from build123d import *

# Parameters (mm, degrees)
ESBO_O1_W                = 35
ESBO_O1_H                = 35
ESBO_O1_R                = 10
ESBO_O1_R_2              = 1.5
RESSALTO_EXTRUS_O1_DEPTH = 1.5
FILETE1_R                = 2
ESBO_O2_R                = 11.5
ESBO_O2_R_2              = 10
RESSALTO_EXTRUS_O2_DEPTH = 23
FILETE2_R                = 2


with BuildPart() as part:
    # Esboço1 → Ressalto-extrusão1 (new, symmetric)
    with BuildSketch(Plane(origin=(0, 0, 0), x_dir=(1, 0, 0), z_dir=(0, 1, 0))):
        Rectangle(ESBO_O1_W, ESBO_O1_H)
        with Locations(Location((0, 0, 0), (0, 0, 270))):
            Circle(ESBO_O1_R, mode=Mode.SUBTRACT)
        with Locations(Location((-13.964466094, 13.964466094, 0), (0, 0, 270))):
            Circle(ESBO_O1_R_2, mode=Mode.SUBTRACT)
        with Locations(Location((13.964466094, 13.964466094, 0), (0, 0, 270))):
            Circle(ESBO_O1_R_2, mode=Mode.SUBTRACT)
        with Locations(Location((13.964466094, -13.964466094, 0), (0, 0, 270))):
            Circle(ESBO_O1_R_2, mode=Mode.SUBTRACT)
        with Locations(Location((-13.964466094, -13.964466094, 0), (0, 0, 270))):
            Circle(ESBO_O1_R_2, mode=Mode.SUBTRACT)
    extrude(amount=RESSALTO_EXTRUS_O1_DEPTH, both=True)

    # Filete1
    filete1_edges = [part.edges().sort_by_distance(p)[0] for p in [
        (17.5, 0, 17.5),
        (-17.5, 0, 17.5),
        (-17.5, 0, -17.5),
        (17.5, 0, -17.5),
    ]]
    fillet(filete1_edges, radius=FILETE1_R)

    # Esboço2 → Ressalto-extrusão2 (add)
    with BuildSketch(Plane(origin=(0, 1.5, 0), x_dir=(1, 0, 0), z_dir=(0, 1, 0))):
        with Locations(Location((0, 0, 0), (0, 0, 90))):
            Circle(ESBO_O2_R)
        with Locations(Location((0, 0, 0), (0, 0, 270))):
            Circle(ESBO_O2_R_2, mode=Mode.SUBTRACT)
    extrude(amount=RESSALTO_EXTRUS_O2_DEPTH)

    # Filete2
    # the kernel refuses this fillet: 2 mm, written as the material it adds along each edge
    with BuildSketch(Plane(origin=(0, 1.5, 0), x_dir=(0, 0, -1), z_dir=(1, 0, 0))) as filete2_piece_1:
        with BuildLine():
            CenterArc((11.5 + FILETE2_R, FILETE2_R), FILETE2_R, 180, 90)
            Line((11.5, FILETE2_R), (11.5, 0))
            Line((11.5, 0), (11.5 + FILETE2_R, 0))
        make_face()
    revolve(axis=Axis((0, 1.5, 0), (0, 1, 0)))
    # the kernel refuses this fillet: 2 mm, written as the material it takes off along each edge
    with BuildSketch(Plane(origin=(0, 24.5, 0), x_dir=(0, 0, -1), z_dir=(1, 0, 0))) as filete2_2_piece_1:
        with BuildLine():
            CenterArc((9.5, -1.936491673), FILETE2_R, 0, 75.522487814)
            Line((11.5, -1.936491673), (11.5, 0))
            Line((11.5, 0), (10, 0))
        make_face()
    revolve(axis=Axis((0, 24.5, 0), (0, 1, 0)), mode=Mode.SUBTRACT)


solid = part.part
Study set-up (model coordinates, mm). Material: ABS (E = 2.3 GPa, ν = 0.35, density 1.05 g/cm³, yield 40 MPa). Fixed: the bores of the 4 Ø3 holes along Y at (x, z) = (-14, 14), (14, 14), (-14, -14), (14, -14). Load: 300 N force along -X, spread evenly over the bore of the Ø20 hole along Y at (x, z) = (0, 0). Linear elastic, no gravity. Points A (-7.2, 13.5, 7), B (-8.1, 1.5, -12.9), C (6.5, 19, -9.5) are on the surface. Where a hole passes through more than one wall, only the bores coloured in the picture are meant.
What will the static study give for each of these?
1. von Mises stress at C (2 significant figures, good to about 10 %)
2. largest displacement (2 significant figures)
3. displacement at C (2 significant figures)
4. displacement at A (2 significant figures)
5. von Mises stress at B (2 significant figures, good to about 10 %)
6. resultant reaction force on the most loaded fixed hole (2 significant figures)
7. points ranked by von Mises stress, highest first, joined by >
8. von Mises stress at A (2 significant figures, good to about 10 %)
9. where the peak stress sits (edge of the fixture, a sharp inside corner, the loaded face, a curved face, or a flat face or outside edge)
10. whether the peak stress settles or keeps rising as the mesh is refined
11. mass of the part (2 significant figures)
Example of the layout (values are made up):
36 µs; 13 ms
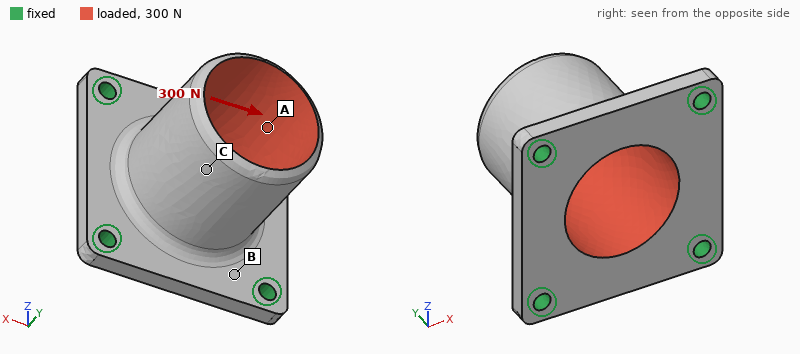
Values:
1.8 MPa; 0.39 mm; 0.29 mm; 0.22 mm; 6.9 MPa; 110 N; B > A > C; 3.9 MPa; edge of the fixture; keeps rising; 5.2 g
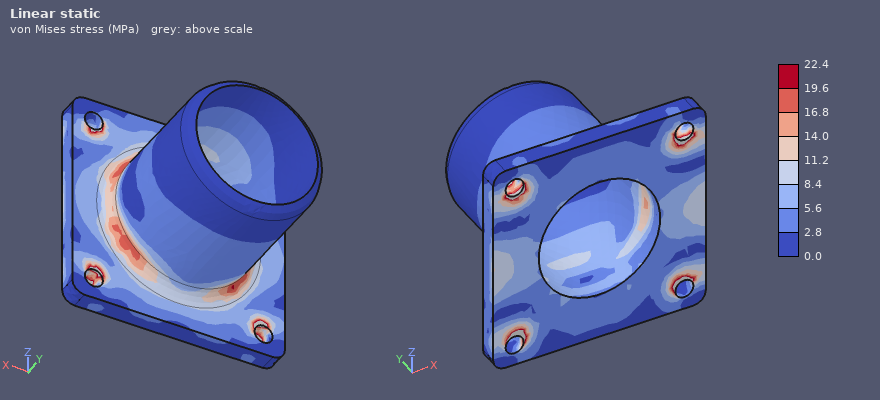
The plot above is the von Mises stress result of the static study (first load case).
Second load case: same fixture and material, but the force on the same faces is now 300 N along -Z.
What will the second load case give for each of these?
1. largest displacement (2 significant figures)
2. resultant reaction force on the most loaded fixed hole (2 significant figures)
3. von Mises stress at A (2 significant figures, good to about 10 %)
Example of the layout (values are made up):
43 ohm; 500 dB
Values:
0.39 mm; 110 N; 4.0 MPa
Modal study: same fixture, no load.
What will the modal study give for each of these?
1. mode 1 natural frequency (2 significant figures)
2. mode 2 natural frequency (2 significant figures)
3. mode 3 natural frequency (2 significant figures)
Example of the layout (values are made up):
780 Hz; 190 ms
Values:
3000 Hz; 3000 Hz; 3100 Hz
